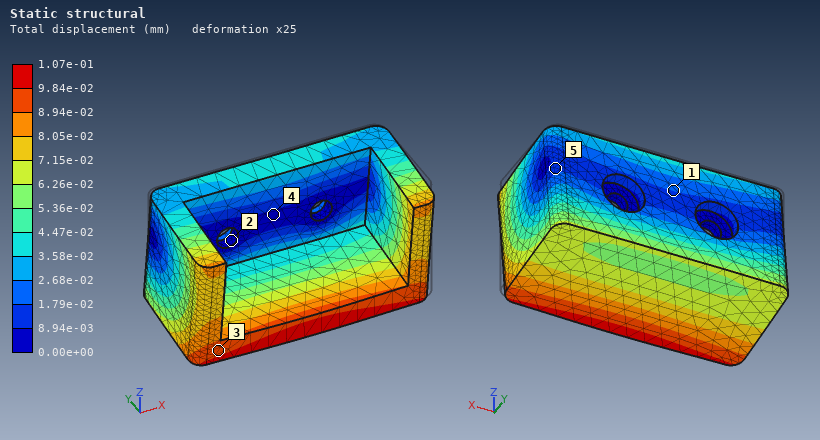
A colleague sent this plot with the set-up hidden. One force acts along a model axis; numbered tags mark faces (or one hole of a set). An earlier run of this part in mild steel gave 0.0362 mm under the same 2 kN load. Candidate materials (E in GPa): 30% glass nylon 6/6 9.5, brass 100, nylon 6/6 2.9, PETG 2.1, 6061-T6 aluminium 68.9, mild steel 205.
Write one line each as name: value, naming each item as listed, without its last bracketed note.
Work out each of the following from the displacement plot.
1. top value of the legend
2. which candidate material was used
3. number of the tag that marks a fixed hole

top value of the legend: 1.07e-01 mm
which candidate material was used: 6061-T6 aluminium
number of the tag that marks a fixed hole: 2
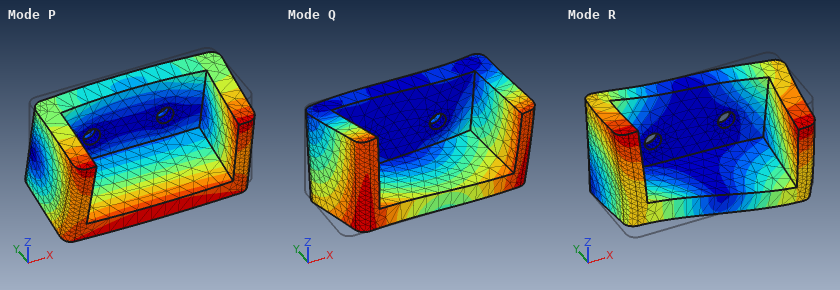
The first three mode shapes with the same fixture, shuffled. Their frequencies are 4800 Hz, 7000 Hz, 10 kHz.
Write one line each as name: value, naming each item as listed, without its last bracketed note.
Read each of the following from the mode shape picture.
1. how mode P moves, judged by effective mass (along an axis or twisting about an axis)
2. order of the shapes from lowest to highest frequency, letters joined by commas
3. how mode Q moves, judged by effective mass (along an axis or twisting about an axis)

how mode P moves, judged by effective mass: along Z
order of the shapes from lowest to highest frequency, letters joined by commas: P, Q, R
how mode Q moves, judged by effective mass: along X
